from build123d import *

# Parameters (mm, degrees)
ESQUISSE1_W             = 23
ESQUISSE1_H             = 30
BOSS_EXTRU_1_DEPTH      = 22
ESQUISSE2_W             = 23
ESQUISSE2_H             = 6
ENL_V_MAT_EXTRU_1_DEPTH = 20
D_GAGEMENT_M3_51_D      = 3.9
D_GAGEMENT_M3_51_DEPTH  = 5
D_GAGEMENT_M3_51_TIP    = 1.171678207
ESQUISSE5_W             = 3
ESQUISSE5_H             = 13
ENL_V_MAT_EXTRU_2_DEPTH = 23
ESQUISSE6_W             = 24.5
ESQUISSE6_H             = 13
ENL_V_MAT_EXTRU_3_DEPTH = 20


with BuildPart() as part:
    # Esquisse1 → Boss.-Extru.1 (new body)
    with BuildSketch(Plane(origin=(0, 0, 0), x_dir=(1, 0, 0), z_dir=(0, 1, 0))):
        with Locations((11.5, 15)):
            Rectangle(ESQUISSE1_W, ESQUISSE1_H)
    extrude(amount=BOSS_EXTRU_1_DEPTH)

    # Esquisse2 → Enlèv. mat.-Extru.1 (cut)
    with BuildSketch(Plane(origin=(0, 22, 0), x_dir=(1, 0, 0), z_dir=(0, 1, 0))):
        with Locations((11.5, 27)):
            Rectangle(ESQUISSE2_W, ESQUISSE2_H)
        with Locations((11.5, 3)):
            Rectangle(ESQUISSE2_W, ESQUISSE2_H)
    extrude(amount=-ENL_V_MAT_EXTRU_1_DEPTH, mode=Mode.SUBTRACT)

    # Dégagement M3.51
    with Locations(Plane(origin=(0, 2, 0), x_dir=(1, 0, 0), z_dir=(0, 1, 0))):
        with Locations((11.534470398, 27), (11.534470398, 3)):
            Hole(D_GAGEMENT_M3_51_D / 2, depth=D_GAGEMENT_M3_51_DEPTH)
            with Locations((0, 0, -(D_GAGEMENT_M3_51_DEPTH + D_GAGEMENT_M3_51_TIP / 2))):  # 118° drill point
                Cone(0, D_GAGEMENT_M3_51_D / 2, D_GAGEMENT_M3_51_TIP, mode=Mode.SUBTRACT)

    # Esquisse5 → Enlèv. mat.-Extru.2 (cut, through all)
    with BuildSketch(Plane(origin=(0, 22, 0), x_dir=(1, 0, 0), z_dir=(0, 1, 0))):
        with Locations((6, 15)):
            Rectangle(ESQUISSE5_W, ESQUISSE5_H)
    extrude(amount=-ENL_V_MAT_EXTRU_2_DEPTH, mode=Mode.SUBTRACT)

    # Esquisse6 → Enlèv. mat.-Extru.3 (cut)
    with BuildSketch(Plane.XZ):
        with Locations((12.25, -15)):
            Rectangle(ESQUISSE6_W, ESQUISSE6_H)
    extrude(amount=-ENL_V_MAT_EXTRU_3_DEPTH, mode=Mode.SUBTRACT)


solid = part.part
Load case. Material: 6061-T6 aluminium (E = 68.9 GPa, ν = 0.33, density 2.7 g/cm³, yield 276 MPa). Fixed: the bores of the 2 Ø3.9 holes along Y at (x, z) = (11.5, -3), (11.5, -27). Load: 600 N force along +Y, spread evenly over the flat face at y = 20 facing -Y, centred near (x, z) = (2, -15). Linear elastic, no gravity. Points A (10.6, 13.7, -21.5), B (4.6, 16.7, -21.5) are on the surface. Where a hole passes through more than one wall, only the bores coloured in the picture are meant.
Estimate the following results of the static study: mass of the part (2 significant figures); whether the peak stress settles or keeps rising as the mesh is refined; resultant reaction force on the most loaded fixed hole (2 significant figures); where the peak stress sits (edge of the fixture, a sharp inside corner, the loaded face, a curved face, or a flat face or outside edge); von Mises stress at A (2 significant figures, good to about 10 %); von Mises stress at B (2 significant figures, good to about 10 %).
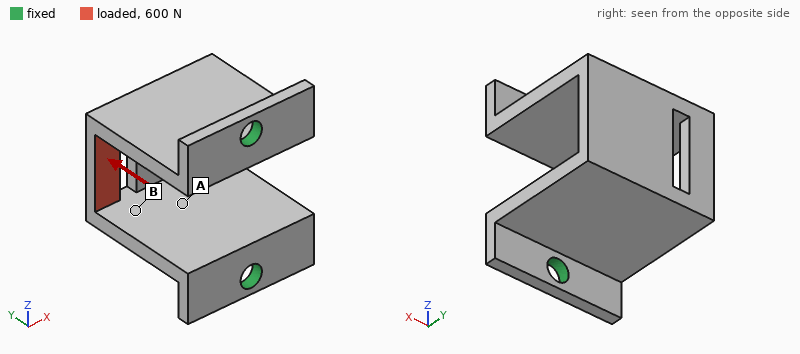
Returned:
9.6 g
keeps rising
310 N
edge of the fixture
19 MPa
57 MPa
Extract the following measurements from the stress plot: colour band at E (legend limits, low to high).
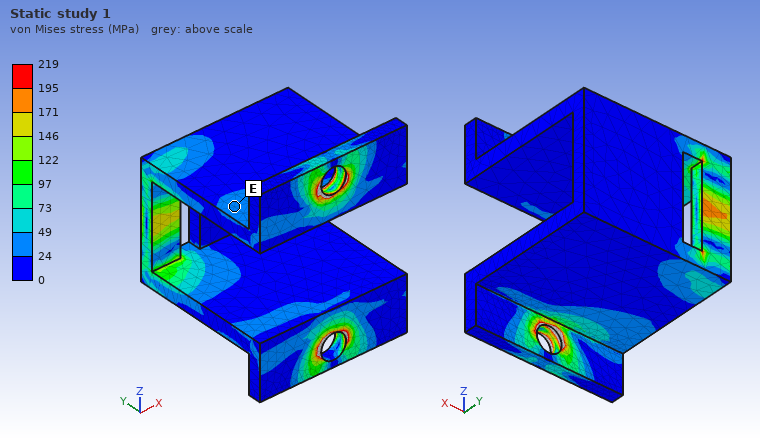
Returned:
24 to 49 MPa
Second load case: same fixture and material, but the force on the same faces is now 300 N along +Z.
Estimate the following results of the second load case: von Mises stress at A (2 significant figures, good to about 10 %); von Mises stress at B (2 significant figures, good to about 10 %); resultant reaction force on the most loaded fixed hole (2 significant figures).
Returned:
35 MPa
54 MPa
250 N
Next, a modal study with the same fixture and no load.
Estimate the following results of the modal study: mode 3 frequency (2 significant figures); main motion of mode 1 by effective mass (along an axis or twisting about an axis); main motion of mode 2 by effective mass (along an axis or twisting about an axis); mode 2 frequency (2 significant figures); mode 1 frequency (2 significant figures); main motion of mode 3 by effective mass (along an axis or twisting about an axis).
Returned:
6200 Hz
along X
along Z
4100 Hz
3700 Hz
twisting about Y
